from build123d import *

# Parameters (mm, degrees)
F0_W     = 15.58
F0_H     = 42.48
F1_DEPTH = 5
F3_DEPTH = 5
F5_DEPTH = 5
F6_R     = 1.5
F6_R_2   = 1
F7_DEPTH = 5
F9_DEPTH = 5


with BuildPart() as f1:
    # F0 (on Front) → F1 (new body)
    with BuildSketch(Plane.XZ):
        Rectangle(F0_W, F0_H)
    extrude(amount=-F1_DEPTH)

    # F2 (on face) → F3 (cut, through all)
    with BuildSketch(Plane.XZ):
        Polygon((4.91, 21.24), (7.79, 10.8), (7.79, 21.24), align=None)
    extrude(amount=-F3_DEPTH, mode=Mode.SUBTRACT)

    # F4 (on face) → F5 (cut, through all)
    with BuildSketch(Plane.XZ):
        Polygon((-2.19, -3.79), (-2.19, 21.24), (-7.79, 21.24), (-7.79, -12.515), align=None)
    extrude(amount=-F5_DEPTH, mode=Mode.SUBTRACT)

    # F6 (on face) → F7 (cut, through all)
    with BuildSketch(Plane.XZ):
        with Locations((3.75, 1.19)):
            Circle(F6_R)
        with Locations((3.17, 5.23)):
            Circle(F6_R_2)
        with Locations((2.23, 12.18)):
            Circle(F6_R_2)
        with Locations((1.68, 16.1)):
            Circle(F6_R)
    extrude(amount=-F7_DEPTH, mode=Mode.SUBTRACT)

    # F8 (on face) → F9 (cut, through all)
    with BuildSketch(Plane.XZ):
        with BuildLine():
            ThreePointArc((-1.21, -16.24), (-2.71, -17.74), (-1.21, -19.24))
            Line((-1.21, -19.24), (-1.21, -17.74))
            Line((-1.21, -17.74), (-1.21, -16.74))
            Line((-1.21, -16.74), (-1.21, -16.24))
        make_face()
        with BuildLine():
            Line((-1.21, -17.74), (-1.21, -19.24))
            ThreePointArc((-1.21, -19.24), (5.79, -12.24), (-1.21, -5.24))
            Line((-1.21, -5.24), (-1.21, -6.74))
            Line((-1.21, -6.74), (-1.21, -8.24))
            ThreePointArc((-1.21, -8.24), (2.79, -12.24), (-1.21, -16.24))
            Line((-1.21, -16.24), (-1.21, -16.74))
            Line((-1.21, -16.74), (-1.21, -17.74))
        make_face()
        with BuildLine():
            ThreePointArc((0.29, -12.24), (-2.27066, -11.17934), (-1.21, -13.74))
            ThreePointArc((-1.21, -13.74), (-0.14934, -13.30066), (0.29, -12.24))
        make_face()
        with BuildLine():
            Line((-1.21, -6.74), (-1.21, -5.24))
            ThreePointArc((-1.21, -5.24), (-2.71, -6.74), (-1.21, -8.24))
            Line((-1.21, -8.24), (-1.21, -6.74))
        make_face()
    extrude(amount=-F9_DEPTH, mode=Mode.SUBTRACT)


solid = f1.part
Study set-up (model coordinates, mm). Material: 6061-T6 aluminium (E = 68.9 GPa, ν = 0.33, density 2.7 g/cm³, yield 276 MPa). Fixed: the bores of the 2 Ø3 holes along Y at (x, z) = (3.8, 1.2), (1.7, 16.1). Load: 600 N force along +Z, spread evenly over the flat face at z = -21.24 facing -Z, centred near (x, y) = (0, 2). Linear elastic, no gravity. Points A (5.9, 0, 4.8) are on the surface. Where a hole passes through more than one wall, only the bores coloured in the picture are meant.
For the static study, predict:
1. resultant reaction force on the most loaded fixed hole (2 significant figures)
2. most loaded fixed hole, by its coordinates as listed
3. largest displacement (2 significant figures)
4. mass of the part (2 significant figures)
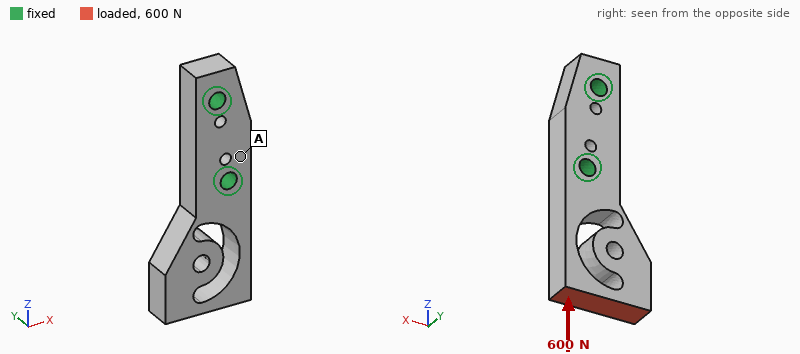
490 N
(3.8, 1.2)
51 µm
5.3 g
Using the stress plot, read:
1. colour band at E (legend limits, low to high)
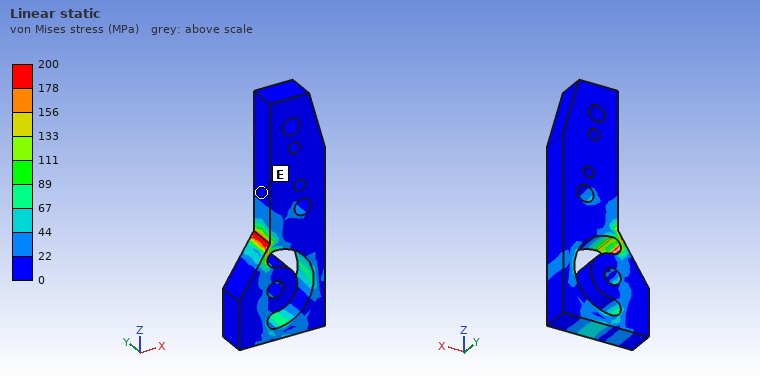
0 to 22 MPa
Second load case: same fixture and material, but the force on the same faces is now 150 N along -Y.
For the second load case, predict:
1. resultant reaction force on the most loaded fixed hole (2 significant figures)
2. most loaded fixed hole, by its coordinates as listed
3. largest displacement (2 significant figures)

190 N
(3.8, 1.2)
0.17 mm
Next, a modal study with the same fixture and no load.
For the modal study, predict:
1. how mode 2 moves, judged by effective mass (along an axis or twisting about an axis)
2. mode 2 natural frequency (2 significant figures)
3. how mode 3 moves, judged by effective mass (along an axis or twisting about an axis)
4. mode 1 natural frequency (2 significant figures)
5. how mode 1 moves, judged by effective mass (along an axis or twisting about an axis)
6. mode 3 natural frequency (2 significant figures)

along X
6700 Hz
twisting about Z
5200 Hz
along Y
12 kHz
